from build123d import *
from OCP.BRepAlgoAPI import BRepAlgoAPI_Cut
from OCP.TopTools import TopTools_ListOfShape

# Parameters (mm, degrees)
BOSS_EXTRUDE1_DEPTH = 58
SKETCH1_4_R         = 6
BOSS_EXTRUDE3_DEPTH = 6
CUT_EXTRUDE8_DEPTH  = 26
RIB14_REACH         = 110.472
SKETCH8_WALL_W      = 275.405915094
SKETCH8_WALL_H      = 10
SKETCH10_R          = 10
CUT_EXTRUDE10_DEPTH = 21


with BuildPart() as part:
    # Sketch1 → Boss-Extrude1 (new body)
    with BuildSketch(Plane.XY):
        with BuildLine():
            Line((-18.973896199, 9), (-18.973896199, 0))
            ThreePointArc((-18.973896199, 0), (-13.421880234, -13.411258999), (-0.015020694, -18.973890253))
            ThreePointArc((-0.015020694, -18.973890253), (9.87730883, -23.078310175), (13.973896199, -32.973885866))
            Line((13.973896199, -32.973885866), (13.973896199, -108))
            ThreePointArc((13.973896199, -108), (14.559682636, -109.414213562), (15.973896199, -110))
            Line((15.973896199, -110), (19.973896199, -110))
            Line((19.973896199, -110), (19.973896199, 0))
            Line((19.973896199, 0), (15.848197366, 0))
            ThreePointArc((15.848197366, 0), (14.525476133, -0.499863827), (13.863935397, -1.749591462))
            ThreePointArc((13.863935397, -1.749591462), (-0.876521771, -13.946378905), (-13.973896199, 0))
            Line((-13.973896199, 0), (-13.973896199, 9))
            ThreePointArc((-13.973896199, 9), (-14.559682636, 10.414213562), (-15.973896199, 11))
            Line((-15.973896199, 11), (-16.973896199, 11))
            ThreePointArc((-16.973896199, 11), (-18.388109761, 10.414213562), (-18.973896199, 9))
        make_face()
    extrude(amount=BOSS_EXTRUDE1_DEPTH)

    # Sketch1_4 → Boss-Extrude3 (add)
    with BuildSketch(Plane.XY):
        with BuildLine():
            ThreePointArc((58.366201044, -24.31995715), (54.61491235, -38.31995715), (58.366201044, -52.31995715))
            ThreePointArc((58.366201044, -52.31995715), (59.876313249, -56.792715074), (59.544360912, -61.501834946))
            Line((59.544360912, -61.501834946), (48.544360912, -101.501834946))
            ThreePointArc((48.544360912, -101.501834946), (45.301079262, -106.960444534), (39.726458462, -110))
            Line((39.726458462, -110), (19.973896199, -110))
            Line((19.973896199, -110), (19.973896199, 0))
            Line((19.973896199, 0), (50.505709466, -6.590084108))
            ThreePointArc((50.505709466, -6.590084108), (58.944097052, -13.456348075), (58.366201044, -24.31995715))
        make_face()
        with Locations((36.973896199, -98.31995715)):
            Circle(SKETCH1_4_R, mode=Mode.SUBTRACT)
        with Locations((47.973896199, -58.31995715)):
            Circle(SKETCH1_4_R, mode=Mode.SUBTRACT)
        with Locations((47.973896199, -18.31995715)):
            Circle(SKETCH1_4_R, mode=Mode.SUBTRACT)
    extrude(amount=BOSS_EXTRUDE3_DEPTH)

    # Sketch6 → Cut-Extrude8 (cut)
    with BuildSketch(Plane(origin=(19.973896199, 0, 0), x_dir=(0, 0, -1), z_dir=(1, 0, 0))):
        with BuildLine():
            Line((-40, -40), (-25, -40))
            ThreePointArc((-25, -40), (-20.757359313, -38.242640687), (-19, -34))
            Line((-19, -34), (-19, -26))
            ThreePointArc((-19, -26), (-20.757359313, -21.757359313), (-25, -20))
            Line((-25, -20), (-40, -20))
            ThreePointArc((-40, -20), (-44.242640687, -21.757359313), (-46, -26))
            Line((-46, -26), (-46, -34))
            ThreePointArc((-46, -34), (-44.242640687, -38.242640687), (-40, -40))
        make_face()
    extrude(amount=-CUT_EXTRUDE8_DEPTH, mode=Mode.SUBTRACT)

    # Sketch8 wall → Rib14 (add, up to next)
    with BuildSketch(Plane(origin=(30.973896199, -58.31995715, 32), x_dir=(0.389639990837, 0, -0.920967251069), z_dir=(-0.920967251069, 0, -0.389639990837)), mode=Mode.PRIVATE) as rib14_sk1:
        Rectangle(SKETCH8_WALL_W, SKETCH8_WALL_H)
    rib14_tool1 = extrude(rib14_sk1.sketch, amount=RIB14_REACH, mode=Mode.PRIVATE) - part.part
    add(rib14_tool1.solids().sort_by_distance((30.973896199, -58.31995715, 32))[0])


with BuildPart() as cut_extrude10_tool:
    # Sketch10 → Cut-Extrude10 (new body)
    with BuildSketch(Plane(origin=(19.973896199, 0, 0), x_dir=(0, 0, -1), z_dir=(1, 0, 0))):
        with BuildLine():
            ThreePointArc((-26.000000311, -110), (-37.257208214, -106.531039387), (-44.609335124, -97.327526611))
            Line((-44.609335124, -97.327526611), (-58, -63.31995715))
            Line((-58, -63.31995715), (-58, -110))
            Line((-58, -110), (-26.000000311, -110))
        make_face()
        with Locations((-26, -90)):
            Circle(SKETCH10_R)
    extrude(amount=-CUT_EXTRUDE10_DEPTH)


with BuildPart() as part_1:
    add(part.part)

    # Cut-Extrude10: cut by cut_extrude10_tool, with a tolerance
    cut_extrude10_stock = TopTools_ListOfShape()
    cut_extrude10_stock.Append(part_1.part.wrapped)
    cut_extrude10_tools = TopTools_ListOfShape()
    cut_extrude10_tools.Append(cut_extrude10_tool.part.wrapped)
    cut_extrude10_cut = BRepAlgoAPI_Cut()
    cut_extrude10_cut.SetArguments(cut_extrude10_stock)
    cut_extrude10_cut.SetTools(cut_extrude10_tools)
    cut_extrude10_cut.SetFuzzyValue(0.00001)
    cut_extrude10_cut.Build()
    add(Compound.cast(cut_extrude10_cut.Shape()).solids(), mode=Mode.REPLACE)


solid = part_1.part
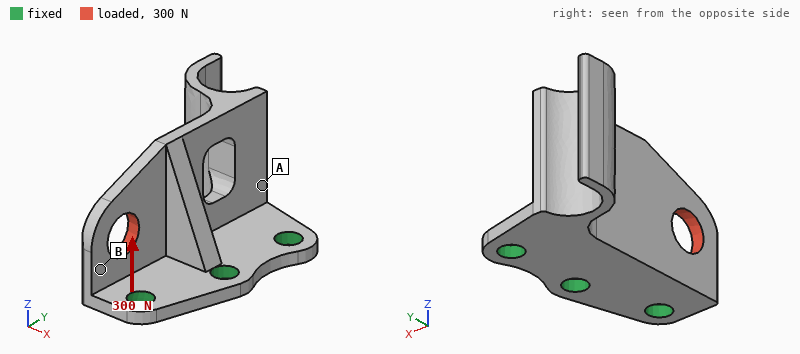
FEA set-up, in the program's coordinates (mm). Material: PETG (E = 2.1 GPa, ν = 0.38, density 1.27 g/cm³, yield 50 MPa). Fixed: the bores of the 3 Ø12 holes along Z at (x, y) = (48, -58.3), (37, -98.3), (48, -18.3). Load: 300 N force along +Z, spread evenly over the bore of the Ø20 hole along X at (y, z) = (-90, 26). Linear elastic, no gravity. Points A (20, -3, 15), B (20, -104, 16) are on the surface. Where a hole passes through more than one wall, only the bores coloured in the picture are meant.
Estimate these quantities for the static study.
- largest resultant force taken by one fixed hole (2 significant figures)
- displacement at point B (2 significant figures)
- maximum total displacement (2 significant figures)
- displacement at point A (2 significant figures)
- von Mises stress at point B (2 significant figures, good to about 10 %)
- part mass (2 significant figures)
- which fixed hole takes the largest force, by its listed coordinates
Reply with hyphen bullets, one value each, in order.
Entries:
- 260 N
- 0.30 mm
- 0.58 mm
- 0.10 mm
- 4.1 MPa
- 96 g
- (37, -98.3)
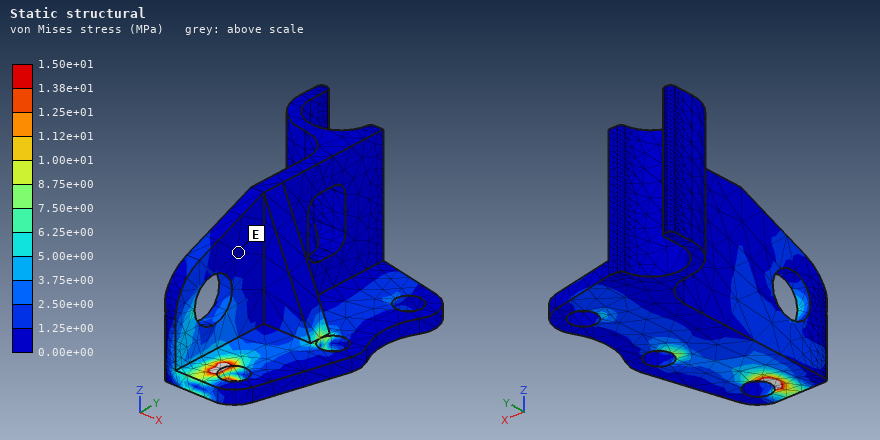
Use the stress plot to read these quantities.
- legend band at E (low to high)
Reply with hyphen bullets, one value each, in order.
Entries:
- 0.00e+00 to 1.25e+00 MPa
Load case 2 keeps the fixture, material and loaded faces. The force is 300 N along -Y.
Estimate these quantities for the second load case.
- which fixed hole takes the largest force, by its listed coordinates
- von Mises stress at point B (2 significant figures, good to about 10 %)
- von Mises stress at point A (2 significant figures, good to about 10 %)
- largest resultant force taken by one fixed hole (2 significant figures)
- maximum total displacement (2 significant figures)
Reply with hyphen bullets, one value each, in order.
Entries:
- (37, -98.3)
- 2.2 MPa
- 0.74 MPa
- 180 N
- 0.52 mm
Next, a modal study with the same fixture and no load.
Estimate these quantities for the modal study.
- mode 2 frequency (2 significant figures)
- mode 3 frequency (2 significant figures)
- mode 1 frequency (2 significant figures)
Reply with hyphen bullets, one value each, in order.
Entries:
- 500 Hz
- 750 Hz
- 230 Hz
